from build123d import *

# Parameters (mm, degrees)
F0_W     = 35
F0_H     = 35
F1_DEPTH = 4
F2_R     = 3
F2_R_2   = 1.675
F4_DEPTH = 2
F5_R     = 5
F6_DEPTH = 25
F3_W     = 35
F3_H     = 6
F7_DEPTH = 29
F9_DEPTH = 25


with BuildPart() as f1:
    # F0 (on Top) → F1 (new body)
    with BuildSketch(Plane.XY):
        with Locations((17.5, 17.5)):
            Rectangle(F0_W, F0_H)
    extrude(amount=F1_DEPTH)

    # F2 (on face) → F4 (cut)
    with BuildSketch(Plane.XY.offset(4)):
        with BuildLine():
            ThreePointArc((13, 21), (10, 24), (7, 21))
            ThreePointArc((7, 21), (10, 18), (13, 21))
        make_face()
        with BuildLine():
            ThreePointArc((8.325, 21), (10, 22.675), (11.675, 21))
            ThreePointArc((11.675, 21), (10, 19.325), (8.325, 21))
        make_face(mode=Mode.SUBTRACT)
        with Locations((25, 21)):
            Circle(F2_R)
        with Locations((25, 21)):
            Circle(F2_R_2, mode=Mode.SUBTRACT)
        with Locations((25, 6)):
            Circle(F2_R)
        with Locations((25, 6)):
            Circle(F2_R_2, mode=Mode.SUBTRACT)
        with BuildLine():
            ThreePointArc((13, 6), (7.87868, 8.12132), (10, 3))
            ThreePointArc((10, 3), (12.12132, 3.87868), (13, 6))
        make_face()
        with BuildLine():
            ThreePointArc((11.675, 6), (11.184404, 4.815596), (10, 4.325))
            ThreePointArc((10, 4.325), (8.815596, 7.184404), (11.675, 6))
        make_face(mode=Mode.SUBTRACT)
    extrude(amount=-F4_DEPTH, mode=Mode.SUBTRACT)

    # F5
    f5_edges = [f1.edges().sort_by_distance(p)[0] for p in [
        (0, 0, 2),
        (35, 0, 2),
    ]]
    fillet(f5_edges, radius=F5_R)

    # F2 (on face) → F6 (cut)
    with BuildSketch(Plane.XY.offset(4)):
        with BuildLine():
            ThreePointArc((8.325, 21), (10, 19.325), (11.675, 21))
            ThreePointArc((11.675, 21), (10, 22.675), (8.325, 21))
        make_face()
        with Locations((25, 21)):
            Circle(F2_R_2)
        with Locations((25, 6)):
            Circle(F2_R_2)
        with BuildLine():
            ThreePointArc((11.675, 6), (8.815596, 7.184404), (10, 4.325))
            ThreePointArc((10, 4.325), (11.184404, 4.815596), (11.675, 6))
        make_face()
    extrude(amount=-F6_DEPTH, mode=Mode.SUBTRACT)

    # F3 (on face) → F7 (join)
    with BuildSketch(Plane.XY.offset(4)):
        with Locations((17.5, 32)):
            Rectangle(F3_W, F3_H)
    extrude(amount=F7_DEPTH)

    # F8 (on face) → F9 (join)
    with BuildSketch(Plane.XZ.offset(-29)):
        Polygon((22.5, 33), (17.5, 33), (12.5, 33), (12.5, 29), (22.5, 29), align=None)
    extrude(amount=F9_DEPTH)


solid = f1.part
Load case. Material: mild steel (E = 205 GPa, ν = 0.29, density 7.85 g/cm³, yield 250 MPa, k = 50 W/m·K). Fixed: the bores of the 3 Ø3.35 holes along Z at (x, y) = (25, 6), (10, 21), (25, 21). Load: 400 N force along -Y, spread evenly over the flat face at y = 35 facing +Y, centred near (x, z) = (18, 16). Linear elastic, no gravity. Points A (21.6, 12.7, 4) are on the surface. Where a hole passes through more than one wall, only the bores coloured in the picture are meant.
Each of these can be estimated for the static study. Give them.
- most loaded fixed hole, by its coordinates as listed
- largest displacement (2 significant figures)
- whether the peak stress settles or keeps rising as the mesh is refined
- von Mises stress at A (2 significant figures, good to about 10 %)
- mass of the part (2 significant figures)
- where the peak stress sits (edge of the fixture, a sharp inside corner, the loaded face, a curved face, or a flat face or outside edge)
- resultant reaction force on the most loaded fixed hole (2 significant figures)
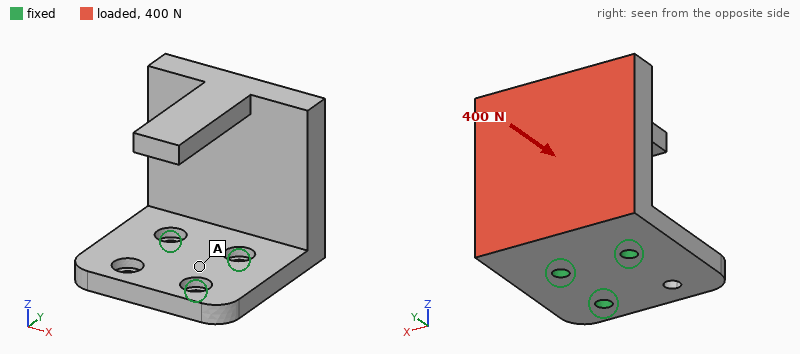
(25, 6)
93 µm
keeps rising
22 MPa
91 g
edge of the fixture
450 N
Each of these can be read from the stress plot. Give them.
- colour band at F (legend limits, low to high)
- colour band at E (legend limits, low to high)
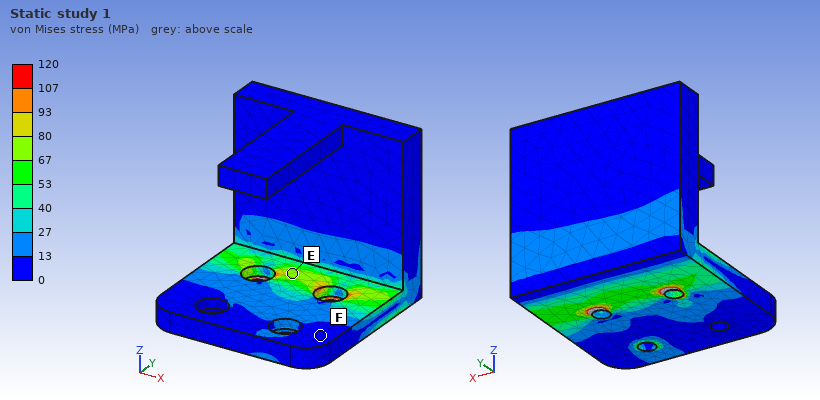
0 to 13 MPa
67 to 80 MPa
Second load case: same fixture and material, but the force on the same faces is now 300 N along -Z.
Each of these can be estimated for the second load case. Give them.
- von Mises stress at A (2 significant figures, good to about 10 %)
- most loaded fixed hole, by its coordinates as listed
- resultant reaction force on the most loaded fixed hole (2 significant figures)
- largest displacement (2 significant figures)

13 MPa
(25, 21)
310 N
44 µm
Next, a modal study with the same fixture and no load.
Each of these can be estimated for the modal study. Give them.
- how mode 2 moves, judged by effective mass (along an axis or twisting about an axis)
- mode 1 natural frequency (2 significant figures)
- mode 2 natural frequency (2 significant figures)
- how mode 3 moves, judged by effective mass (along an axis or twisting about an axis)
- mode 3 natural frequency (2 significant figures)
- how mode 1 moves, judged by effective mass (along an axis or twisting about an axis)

along X
1500 Hz
3000 Hz
along Z
4100 Hz
along Y
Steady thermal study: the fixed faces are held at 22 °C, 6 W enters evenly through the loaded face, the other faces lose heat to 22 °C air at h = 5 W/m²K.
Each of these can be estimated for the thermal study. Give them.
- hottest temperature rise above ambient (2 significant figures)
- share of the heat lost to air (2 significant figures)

19 K
4.0 %
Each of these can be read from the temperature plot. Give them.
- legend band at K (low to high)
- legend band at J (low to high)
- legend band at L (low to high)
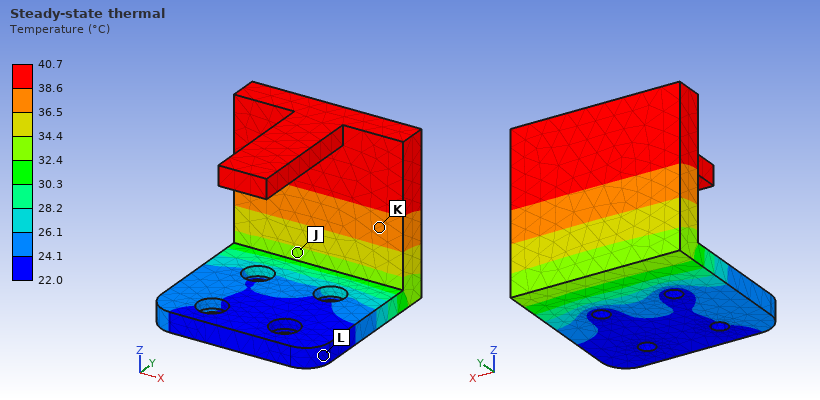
36.5 to 38.6 °C
32.4 to 34.4 °C
22.0 to 24.1 °C
